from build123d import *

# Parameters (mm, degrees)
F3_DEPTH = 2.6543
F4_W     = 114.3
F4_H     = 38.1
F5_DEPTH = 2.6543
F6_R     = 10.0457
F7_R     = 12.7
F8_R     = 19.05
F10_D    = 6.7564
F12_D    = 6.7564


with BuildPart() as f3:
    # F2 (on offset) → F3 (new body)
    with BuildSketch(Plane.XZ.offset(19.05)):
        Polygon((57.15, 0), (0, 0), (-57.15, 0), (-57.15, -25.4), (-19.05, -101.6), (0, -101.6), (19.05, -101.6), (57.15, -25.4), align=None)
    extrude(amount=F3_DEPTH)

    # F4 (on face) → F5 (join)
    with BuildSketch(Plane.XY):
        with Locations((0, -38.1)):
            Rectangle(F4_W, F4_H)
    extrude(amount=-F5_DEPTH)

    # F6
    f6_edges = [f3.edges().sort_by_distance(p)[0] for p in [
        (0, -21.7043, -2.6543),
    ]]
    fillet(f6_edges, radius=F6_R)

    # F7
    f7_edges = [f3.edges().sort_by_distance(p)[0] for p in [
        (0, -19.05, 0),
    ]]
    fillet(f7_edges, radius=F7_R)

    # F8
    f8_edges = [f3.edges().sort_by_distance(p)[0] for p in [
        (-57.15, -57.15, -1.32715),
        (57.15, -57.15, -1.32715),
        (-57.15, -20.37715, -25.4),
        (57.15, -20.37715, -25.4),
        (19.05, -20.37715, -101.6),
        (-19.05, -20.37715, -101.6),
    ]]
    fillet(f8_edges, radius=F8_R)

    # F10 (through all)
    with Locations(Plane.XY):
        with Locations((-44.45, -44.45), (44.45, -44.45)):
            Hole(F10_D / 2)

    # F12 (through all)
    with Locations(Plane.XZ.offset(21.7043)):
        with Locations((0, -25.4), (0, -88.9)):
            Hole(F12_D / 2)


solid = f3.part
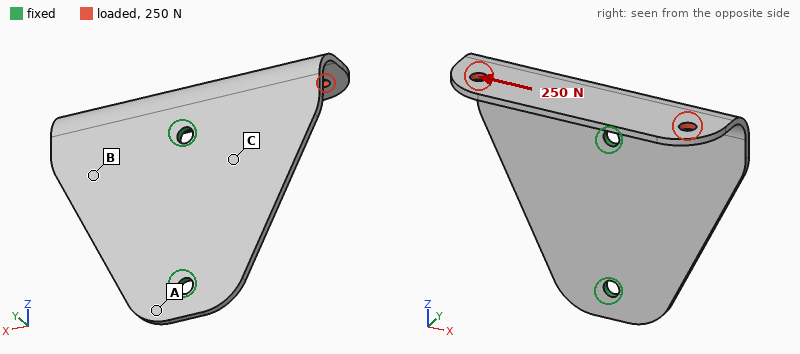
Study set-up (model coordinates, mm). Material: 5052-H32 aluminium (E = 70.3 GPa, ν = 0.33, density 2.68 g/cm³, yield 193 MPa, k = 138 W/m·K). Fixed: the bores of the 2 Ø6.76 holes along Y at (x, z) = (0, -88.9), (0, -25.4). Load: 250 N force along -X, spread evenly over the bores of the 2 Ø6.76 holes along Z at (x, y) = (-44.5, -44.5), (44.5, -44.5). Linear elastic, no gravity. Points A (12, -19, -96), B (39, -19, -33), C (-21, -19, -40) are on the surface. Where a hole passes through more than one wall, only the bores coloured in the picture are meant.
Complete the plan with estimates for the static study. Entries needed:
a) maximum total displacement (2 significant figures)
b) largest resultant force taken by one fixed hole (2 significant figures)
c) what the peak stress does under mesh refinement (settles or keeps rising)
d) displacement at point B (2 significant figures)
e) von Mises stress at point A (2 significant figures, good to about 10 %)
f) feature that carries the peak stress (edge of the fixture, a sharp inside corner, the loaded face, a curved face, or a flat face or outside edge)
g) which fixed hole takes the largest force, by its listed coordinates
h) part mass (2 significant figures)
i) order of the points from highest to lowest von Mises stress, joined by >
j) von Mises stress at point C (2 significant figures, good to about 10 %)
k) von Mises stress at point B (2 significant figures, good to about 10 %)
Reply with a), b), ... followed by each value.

a) 0.54 mm
b) 330 N
c) keeps rising
d) 0.19 mm
e) 6.3 MPa
f) edge of the fixture
g) (0, -25.4)
h) 84 g
i) C > B > A
j) 21 MPa
k) 13 MPa
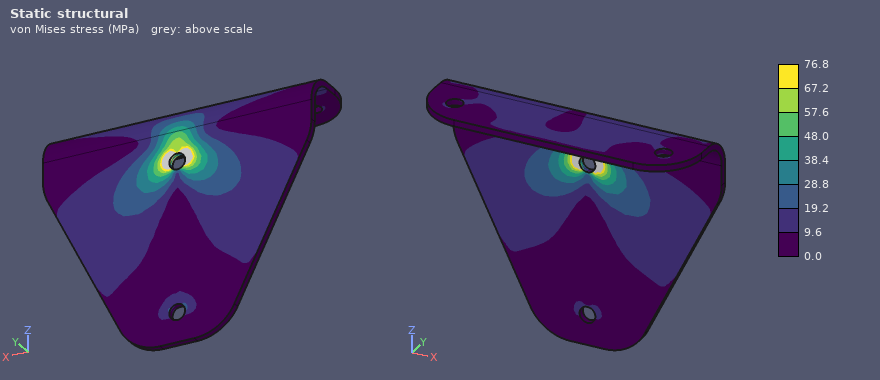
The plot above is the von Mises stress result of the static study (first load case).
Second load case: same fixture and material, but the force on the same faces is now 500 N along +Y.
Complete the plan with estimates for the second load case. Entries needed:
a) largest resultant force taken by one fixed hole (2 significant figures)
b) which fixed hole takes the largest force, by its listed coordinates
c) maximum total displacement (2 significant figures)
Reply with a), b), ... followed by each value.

a) 580 N
b) (0, -25.4)
c) 0.71 mm
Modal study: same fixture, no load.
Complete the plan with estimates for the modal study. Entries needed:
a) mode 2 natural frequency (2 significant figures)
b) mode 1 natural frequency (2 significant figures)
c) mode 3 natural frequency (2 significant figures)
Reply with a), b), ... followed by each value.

a) 750 Hz
b) 550 Hz
c) 1300 Hz
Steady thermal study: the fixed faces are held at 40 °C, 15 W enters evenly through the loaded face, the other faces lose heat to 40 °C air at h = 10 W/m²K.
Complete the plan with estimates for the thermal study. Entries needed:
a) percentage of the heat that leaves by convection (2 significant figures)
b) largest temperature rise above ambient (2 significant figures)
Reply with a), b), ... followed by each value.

a) 18 %
b) 30 K
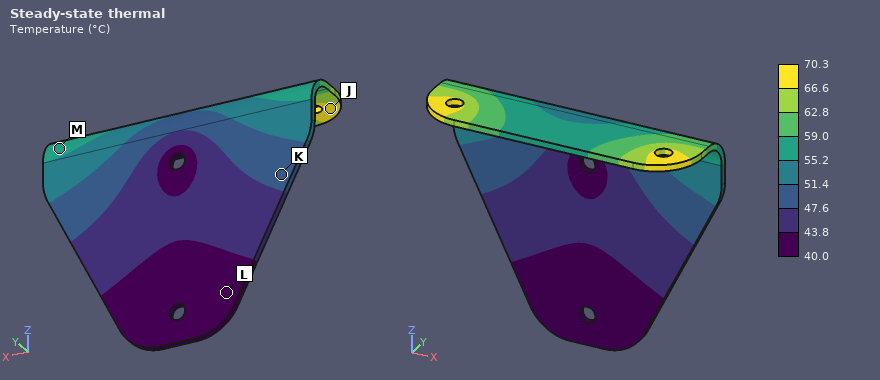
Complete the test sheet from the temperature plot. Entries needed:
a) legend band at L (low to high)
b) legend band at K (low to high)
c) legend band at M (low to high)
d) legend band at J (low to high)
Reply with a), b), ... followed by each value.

a) 40.0 to 43.8 °C
b) 47.6 to 51.4 °C
c) 55.2 to 59.0 °C
d) 66.6 to 70.3 °C
